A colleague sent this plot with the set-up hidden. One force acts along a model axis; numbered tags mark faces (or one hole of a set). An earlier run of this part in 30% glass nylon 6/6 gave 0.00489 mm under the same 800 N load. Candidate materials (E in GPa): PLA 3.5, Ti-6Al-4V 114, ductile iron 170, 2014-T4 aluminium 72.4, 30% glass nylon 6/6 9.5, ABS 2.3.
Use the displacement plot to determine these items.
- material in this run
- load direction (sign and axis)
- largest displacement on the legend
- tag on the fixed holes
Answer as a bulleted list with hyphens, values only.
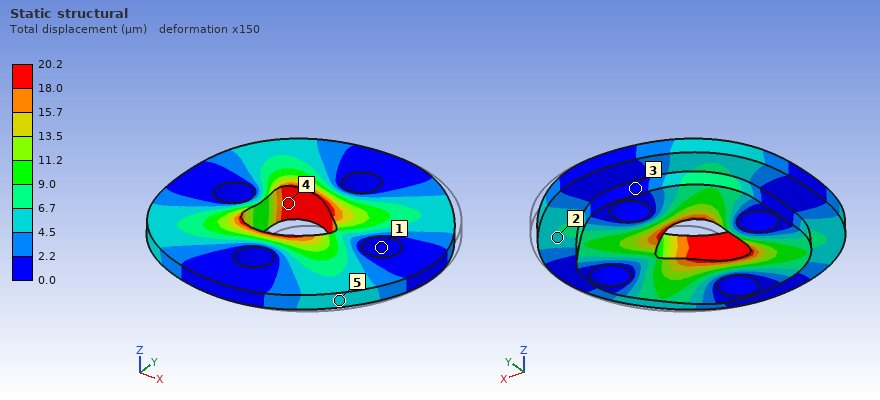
- ABS
- -X
- 20.2 µm
- 1
